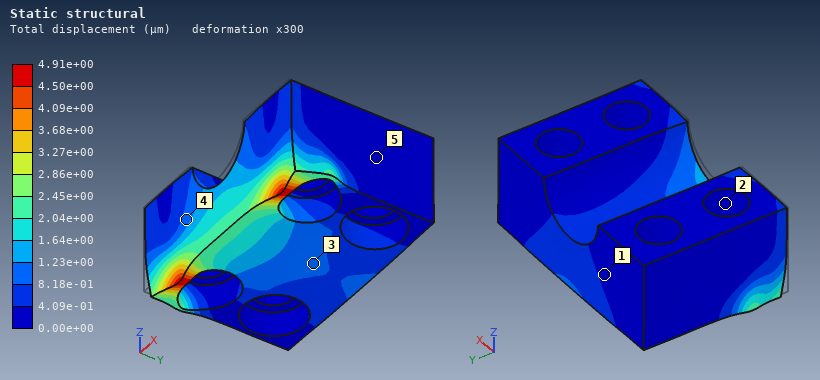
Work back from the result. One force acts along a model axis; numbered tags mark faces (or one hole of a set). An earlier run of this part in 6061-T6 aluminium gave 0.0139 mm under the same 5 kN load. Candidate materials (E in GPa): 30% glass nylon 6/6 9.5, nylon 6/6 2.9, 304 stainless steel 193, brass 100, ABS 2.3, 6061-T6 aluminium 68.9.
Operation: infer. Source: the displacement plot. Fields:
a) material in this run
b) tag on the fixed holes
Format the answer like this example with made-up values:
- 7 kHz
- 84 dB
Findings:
- 304 stainless steel
- 2
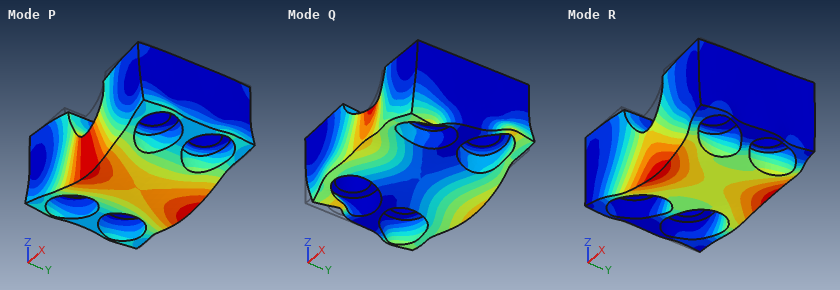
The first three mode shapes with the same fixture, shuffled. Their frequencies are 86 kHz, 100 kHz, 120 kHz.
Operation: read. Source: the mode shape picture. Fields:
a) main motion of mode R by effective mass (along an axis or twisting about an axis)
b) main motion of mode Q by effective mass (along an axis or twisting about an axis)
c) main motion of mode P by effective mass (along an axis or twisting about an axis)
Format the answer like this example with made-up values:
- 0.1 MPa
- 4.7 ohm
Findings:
- along Y
- along Y
- along Z
